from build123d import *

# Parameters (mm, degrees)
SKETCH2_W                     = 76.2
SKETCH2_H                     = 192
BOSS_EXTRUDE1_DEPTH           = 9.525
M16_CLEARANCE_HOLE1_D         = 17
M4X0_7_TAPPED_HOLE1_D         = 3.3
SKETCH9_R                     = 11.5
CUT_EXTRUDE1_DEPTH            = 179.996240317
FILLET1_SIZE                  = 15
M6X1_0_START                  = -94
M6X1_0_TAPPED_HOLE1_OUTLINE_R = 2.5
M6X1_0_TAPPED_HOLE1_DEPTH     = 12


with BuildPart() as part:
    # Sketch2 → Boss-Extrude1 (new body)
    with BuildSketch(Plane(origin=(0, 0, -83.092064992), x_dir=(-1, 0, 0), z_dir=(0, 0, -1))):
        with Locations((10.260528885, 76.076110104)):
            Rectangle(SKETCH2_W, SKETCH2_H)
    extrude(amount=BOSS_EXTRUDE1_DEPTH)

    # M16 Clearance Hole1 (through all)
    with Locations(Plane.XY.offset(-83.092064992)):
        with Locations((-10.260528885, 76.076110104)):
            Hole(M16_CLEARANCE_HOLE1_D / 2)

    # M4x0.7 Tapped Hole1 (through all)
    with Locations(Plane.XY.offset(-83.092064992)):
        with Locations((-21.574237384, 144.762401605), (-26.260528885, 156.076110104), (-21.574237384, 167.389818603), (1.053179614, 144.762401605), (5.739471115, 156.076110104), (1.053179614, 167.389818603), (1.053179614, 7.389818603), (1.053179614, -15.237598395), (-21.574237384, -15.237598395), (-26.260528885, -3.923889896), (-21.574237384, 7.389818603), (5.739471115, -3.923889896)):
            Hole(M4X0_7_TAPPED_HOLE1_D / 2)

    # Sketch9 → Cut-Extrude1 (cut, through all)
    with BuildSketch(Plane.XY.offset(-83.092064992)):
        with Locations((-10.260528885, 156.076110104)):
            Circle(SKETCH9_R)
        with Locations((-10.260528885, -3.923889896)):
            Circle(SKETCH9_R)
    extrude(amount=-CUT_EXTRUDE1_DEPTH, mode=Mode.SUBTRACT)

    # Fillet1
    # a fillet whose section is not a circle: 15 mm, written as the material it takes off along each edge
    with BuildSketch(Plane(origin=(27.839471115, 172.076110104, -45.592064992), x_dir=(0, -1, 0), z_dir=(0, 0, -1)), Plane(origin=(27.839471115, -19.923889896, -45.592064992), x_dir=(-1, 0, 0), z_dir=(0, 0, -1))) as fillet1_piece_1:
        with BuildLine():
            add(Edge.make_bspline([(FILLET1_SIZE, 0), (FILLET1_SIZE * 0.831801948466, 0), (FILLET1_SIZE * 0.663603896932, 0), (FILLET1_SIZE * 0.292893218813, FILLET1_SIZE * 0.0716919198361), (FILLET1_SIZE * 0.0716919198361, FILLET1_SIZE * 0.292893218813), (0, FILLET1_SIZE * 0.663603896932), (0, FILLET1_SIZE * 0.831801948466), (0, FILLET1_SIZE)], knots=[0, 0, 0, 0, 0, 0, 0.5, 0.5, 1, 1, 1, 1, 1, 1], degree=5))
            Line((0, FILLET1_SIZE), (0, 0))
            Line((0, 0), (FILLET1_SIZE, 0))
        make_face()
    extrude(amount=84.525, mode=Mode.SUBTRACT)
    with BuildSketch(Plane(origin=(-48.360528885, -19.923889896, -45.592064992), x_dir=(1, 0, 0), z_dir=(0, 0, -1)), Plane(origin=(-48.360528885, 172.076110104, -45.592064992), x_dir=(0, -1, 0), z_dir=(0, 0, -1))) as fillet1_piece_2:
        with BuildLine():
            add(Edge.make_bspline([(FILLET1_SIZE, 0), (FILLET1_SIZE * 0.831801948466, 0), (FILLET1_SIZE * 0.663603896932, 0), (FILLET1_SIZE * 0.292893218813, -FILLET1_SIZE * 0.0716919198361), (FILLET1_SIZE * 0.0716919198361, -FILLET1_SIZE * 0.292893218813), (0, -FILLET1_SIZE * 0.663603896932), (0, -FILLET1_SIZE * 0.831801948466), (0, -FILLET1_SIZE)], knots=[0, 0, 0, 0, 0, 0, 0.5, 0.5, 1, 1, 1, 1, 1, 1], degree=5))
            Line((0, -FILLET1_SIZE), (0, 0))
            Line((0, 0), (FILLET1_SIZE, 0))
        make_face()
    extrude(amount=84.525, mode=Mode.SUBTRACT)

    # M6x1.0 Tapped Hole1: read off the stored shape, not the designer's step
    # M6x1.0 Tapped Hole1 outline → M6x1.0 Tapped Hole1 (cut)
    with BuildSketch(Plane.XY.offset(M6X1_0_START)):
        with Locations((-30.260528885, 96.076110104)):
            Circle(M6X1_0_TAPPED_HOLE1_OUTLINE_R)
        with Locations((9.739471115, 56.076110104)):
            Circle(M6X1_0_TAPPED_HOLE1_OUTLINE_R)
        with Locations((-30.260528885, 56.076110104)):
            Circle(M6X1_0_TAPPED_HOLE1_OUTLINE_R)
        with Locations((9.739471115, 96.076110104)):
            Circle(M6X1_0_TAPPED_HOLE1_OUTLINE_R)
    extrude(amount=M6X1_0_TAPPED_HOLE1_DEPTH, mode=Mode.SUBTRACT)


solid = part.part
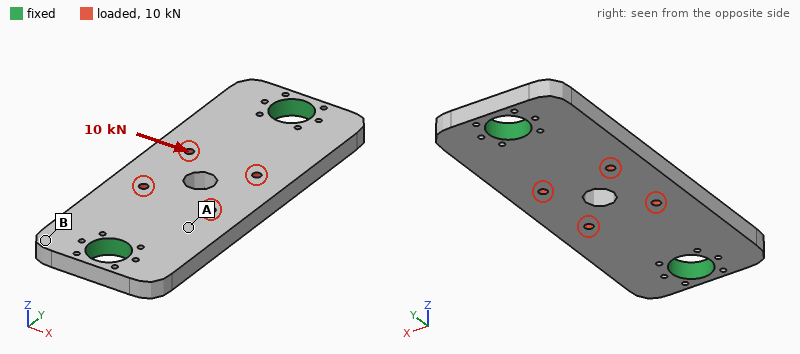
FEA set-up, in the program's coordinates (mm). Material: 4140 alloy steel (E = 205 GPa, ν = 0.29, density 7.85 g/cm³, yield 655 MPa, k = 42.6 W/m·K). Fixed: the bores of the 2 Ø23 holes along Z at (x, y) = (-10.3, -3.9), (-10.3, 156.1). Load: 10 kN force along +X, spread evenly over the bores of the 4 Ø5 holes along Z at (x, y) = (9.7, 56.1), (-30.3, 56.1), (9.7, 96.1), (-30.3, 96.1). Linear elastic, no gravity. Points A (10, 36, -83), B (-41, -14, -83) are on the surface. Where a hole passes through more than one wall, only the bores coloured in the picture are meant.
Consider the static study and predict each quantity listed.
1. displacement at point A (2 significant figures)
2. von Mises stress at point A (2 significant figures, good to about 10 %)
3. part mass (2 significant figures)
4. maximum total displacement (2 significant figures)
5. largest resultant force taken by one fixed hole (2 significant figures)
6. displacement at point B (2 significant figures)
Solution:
6.9 µm
14 MPa
990 g
11 µm
5.0 kN
2.8 µm
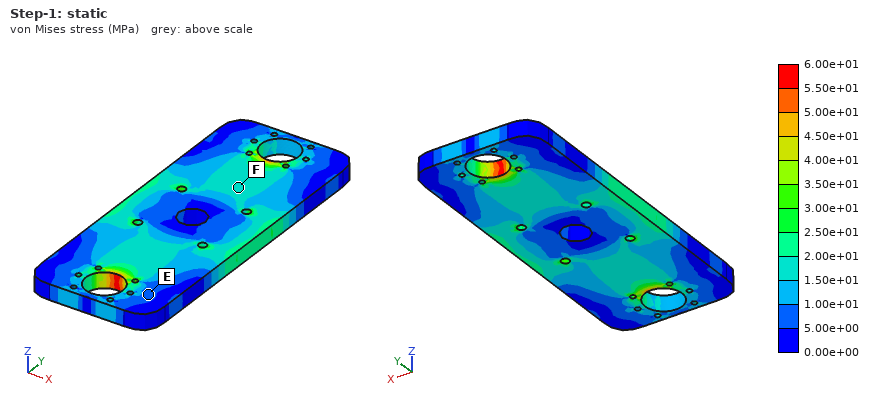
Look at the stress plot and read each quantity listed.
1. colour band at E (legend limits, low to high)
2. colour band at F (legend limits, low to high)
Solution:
5.00e+00 to 1.00e+01 MPa
1.50e+01 to 2.00e+01 MPa
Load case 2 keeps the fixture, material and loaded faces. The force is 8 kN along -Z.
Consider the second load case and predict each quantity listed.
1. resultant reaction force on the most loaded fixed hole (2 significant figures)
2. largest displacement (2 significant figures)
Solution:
4.0 kN
0.12 mm
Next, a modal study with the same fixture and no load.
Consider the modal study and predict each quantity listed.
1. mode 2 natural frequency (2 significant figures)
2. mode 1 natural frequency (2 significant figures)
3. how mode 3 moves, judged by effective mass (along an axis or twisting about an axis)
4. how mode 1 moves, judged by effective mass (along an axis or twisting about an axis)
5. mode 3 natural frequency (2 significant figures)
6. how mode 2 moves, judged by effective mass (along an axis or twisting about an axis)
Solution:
2700 Hz
2100 Hz
twisting about X
along Z
5300 Hz
twisting about Y
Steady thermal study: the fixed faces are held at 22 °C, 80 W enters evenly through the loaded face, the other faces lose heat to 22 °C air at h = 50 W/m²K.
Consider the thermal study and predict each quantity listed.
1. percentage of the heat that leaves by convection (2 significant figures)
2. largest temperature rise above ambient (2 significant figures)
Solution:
49 %
57 K
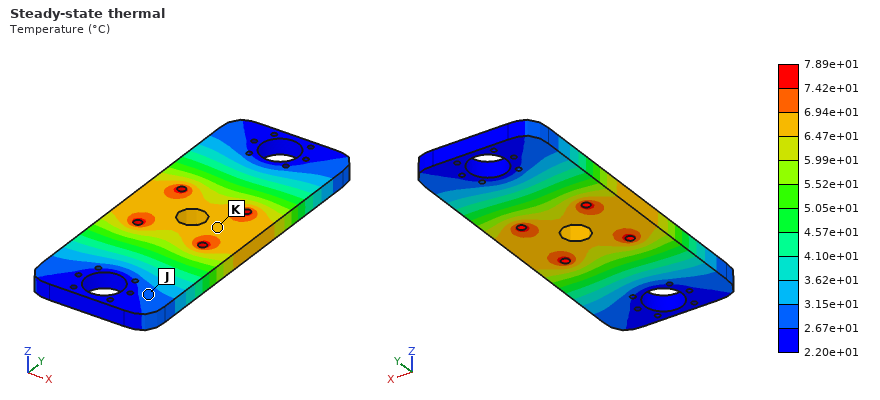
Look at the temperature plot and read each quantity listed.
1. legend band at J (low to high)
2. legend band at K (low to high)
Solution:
2.67e+01 to 3.15e+01 °C
6.47e+01 to 6.94e+01 °C
